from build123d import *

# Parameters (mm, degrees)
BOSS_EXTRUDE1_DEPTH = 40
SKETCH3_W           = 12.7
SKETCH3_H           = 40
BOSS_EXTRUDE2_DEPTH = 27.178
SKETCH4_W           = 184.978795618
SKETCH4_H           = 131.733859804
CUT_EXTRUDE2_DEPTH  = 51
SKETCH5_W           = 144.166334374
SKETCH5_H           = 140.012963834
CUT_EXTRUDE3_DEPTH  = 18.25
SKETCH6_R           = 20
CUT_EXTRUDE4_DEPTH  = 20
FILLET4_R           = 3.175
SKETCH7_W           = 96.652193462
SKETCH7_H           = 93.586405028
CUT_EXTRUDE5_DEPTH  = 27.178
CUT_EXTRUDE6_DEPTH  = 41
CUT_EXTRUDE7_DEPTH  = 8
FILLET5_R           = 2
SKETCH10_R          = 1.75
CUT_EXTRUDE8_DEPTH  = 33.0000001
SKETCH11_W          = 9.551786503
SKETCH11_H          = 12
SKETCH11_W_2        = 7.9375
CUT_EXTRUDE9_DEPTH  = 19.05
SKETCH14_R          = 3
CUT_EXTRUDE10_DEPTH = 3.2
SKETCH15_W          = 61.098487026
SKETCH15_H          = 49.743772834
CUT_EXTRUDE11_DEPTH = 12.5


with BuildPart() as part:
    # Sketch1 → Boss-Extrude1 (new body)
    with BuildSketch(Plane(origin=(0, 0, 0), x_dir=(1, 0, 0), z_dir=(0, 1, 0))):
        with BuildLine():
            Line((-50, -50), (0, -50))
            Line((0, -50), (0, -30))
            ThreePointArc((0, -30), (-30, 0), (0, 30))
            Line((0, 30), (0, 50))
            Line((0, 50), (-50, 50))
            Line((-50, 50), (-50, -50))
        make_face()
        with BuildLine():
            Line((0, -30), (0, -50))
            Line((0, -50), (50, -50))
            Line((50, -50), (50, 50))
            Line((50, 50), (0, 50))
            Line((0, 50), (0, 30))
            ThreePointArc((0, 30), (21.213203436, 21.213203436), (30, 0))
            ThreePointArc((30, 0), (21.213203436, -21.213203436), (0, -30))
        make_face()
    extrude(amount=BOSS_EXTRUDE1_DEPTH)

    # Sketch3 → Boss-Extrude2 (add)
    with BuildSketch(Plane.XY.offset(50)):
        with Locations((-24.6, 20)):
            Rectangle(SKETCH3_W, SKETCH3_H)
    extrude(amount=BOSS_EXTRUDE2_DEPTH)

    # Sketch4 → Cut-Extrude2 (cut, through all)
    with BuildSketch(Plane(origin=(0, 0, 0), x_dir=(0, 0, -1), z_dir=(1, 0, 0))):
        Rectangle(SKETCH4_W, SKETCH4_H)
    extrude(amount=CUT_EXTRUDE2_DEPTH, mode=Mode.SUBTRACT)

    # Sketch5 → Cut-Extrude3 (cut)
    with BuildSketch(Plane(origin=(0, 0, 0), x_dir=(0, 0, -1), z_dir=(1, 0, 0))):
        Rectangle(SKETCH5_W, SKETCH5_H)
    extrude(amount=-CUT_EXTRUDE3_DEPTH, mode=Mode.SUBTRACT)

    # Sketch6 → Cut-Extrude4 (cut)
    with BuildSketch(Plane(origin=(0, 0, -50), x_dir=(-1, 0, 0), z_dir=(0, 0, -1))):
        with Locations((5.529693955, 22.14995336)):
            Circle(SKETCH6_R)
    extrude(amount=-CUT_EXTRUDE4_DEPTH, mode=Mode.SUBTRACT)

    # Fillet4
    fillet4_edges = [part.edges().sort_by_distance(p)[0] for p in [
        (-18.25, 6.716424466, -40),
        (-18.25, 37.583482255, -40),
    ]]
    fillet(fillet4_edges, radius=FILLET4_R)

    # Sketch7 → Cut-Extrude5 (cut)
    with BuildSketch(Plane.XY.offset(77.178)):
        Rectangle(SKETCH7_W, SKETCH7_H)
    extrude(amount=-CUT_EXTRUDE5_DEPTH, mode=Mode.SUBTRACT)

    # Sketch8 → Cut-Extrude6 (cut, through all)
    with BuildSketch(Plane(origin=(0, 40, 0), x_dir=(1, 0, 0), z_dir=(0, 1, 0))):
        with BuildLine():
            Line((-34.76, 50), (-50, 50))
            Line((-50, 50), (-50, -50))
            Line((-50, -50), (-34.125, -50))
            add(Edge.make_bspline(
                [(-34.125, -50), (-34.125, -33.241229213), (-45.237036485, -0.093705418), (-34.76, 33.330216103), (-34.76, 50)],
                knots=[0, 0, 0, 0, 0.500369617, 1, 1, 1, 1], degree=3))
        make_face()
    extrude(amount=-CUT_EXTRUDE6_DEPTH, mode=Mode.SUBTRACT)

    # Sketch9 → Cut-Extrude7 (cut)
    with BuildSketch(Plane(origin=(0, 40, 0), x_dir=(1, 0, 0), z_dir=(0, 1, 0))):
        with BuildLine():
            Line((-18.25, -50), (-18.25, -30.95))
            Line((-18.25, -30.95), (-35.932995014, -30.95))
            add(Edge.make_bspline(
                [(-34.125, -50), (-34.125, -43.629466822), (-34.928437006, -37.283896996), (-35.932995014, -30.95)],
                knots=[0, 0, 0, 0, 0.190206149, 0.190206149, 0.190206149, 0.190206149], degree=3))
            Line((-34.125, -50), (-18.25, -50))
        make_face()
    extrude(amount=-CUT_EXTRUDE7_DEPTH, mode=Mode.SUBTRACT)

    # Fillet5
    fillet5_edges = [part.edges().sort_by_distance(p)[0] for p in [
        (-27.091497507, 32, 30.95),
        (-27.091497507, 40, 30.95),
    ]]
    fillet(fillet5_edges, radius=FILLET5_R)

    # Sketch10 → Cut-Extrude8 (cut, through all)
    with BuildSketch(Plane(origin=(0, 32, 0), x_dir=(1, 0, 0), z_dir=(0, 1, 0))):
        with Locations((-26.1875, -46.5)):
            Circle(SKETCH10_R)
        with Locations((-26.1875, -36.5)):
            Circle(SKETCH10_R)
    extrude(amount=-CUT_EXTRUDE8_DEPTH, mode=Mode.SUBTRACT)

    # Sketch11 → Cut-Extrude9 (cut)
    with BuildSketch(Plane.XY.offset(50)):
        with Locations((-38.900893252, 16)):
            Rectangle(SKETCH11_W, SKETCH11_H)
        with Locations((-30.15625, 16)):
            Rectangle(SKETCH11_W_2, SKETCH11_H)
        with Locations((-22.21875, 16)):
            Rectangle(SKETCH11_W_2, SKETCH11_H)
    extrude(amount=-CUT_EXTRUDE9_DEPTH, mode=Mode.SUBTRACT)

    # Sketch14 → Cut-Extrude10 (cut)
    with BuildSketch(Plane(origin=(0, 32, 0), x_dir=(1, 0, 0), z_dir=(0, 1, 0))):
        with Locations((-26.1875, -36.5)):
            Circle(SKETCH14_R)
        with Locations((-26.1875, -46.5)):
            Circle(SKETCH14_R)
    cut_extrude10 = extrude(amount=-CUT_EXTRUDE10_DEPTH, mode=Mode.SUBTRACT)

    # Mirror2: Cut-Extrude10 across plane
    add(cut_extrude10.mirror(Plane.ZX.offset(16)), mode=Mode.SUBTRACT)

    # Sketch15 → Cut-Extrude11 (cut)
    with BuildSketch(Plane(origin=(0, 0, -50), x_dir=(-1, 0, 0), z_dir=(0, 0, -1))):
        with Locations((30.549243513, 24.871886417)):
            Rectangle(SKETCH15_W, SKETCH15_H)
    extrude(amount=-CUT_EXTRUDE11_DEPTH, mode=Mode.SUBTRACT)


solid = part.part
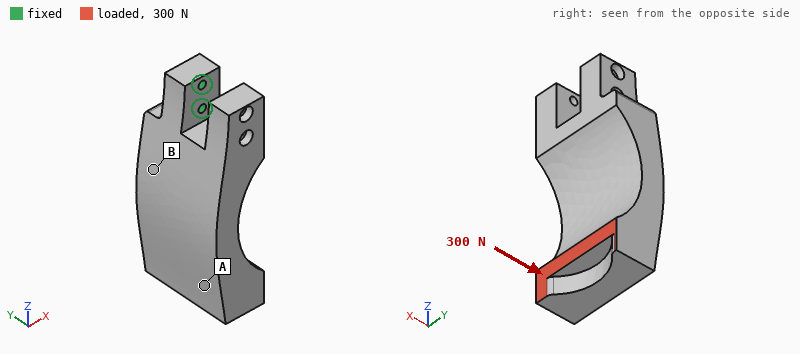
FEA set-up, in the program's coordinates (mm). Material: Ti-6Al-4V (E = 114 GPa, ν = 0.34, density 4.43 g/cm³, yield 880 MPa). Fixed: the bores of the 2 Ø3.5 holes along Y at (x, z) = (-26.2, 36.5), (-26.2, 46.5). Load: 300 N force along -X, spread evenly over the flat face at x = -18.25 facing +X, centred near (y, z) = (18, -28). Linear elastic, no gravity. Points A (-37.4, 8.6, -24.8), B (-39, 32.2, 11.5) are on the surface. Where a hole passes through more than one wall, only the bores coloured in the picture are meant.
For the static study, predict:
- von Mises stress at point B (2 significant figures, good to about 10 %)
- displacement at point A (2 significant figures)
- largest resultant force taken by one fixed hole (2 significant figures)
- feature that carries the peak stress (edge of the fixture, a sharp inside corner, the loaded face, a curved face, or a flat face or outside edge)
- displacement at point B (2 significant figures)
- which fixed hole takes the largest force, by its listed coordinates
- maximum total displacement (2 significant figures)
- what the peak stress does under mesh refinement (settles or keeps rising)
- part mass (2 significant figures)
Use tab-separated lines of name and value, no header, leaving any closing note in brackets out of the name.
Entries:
von Mises stress at point B	15 MPa
displacement at point A	0.078 mm
largest resultant force taken by one fixed hole	1.6 kN
feature that carries the peak stress	edge of the fixture
displacement at point B	0.022 mm
which fixed hole takes the largest force, by its listed coordinates	(-26.2, 36.5)
maximum total displacement	0.10 mm
what the peak stress does under mesh refinement	keeps rising
part mass	190 g
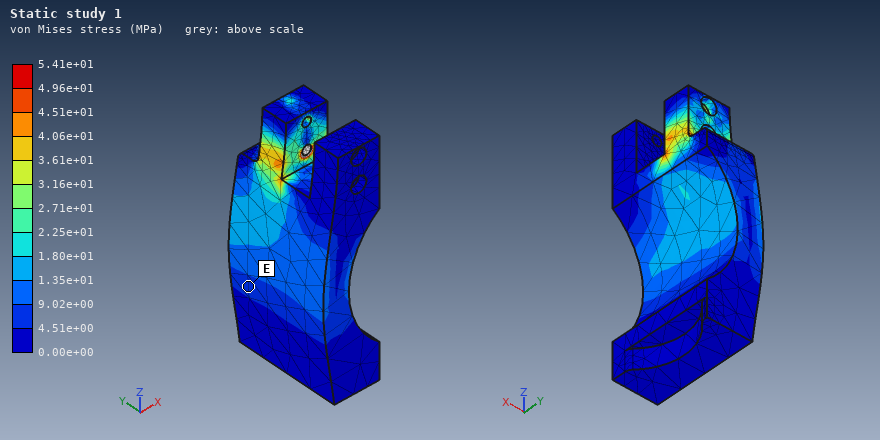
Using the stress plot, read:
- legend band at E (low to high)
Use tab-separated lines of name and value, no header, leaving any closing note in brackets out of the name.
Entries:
legend band at E	4.51e+00 to 9.02e+00 MPa
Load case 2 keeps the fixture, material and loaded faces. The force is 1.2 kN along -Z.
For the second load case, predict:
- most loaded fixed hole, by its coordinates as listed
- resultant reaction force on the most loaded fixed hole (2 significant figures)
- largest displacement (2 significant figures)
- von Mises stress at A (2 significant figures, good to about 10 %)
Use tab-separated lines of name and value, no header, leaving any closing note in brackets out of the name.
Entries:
most loaded fixed hole, by its coordinates as listed	(-26.2, 36.5)
resultant reaction force on the most loaded fixed hole	1.4 kN
largest displacement	0.12 mm
von Mises stress at A	6.8 MPa
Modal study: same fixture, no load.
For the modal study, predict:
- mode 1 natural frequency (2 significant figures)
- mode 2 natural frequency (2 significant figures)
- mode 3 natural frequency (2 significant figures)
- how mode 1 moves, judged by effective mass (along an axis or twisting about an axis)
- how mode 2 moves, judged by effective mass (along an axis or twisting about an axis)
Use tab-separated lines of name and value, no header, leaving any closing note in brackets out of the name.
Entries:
mode 1 natural frequency	930 Hz
mode 2 natural frequency	1100 Hz
mode 3 natural frequency	2800 Hz
how mode 1 moves, judged by effective mass	along Y
how mode 2 moves, judged by effective mass	along X
